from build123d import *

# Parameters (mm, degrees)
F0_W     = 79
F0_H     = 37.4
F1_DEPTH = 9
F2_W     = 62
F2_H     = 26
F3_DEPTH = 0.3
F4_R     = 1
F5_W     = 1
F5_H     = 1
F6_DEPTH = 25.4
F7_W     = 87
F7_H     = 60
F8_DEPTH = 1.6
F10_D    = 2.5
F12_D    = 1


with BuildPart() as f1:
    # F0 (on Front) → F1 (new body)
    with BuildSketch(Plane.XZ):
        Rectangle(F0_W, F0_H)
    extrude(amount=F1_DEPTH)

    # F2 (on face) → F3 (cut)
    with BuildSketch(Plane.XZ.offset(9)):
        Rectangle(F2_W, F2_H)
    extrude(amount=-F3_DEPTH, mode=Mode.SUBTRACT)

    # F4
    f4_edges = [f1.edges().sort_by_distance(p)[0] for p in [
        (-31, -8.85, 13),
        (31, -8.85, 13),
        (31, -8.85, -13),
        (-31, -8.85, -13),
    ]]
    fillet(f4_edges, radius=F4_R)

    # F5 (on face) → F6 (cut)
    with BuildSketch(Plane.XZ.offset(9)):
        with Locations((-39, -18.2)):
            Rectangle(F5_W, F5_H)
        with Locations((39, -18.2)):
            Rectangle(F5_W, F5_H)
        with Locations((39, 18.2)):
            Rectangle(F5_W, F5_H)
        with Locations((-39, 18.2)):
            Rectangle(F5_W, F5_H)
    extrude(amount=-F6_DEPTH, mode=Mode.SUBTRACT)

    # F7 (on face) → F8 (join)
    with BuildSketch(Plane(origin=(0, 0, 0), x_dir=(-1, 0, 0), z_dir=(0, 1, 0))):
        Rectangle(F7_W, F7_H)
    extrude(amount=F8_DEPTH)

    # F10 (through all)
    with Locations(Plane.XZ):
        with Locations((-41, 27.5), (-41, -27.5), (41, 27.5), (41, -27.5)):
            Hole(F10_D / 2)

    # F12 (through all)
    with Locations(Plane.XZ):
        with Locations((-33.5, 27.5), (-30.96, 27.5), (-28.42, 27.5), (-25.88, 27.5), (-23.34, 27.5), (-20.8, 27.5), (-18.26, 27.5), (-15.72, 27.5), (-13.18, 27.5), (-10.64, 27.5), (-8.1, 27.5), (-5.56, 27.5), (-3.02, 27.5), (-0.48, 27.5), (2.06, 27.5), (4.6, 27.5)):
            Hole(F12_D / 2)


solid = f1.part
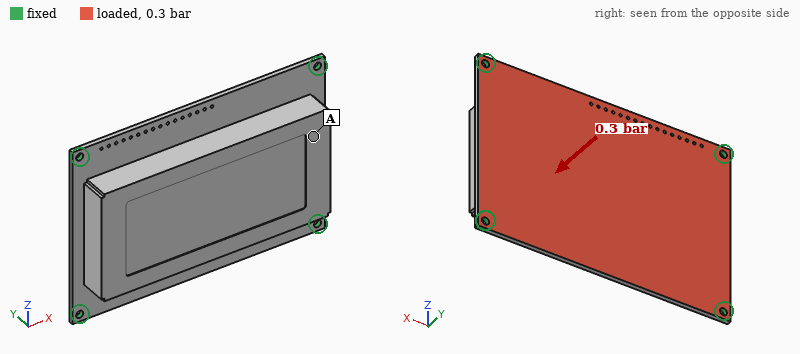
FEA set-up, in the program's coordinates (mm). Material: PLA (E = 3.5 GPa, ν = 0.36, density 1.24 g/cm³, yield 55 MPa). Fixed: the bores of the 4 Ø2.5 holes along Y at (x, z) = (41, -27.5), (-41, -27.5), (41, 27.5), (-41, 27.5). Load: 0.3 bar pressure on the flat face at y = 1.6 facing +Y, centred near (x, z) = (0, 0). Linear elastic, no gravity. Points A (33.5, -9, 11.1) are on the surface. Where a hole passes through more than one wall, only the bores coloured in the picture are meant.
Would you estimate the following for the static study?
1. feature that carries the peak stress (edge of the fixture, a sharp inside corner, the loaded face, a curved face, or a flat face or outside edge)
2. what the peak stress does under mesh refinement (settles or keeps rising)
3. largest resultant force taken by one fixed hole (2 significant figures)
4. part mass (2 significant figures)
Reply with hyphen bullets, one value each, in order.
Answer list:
- edge of the fixture
- keeps rising
- 50 N
- 43 g
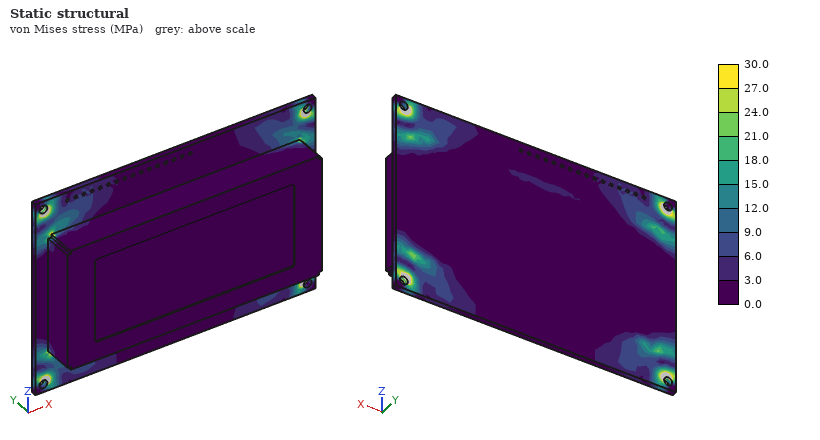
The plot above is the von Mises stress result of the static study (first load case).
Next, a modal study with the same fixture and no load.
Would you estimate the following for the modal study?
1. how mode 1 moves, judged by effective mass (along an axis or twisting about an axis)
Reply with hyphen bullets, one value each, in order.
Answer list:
- along Y
